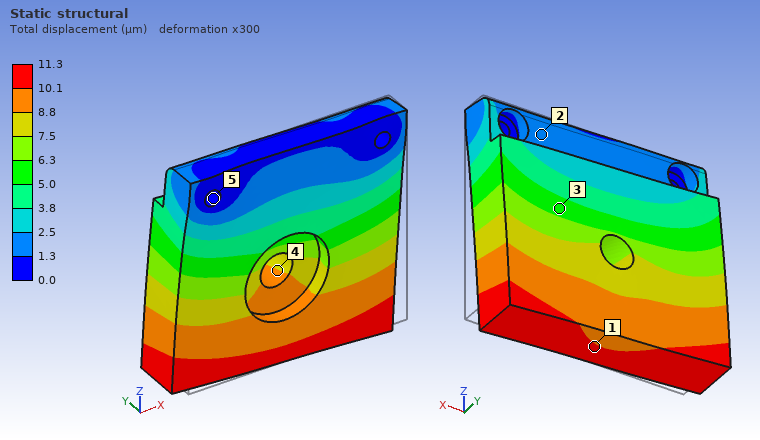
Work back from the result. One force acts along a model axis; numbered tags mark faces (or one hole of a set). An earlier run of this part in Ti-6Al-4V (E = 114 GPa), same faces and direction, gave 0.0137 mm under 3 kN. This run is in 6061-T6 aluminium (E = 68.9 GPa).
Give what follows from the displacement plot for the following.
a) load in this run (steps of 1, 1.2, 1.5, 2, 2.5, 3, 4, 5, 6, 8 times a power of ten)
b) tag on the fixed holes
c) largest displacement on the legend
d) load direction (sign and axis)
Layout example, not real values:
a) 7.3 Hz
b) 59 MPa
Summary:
a) 1.5 kN
b) 5
c) 11.3 µm
d) -X
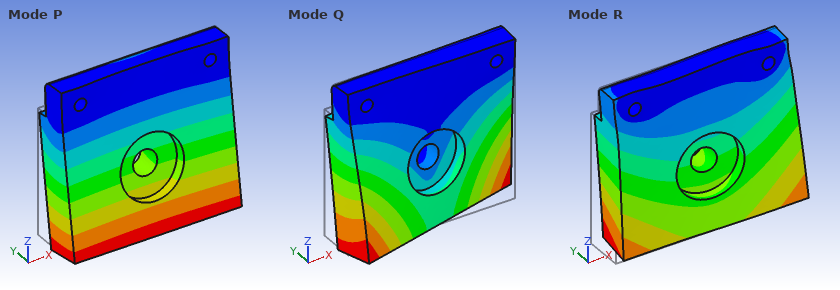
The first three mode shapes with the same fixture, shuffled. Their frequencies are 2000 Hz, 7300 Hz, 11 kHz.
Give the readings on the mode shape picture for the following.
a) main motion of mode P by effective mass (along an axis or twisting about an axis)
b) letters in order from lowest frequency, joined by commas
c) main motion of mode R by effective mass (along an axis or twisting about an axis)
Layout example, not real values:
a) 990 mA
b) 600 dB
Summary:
a) along Y
b) P, Q, R
c) along X
